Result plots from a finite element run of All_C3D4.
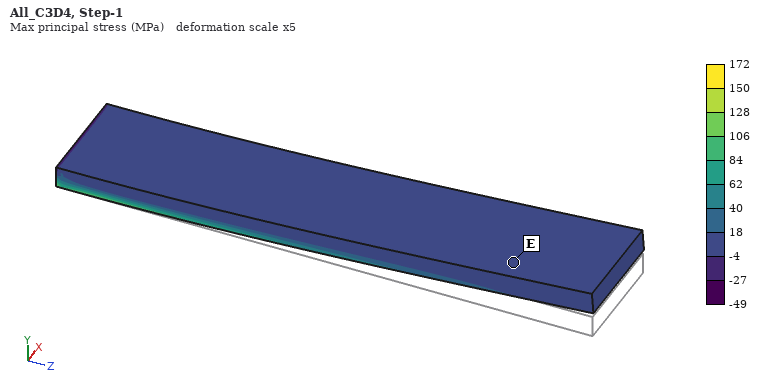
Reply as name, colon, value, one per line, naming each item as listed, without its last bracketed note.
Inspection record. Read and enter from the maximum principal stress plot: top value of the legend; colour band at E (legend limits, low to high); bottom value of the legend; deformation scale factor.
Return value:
top value of the legend: 172 MPa
colour band at E: -4 to 18 MPa
bottom value of the legend: -49 MPa
deformation scale factor: 5
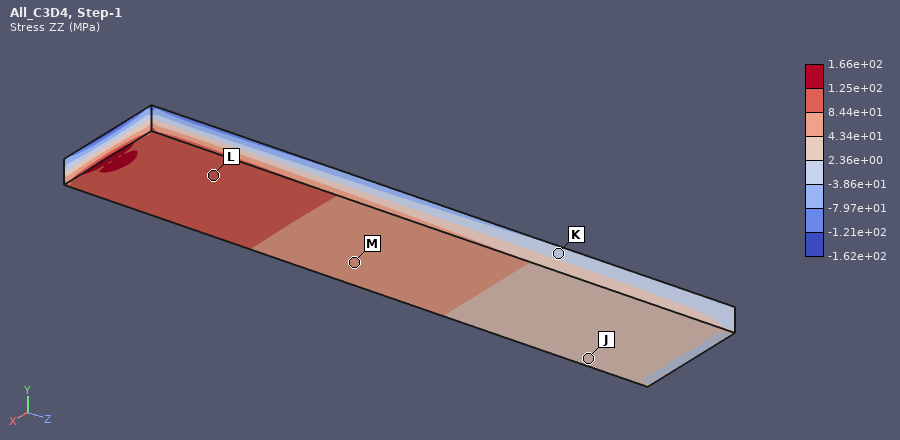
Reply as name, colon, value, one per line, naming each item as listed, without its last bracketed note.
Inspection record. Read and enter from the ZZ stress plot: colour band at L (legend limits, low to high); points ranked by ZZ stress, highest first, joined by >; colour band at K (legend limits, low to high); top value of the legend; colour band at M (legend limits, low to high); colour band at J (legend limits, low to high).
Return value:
colour band at L: 8.44e+01 to 1.25e+02 MPa
points ranked by ZZ stress, highest first, joined by >: L > M > J > K
colour band at K: -3.86e+01 to 2.36e+00 MPa
top value of the legend: 1.66e+02 MPa
colour band at M: 4.34e+01 to 8.44e+01 MPa
colour band at J: 2.36e+00 to 4.34e+01 MPa
